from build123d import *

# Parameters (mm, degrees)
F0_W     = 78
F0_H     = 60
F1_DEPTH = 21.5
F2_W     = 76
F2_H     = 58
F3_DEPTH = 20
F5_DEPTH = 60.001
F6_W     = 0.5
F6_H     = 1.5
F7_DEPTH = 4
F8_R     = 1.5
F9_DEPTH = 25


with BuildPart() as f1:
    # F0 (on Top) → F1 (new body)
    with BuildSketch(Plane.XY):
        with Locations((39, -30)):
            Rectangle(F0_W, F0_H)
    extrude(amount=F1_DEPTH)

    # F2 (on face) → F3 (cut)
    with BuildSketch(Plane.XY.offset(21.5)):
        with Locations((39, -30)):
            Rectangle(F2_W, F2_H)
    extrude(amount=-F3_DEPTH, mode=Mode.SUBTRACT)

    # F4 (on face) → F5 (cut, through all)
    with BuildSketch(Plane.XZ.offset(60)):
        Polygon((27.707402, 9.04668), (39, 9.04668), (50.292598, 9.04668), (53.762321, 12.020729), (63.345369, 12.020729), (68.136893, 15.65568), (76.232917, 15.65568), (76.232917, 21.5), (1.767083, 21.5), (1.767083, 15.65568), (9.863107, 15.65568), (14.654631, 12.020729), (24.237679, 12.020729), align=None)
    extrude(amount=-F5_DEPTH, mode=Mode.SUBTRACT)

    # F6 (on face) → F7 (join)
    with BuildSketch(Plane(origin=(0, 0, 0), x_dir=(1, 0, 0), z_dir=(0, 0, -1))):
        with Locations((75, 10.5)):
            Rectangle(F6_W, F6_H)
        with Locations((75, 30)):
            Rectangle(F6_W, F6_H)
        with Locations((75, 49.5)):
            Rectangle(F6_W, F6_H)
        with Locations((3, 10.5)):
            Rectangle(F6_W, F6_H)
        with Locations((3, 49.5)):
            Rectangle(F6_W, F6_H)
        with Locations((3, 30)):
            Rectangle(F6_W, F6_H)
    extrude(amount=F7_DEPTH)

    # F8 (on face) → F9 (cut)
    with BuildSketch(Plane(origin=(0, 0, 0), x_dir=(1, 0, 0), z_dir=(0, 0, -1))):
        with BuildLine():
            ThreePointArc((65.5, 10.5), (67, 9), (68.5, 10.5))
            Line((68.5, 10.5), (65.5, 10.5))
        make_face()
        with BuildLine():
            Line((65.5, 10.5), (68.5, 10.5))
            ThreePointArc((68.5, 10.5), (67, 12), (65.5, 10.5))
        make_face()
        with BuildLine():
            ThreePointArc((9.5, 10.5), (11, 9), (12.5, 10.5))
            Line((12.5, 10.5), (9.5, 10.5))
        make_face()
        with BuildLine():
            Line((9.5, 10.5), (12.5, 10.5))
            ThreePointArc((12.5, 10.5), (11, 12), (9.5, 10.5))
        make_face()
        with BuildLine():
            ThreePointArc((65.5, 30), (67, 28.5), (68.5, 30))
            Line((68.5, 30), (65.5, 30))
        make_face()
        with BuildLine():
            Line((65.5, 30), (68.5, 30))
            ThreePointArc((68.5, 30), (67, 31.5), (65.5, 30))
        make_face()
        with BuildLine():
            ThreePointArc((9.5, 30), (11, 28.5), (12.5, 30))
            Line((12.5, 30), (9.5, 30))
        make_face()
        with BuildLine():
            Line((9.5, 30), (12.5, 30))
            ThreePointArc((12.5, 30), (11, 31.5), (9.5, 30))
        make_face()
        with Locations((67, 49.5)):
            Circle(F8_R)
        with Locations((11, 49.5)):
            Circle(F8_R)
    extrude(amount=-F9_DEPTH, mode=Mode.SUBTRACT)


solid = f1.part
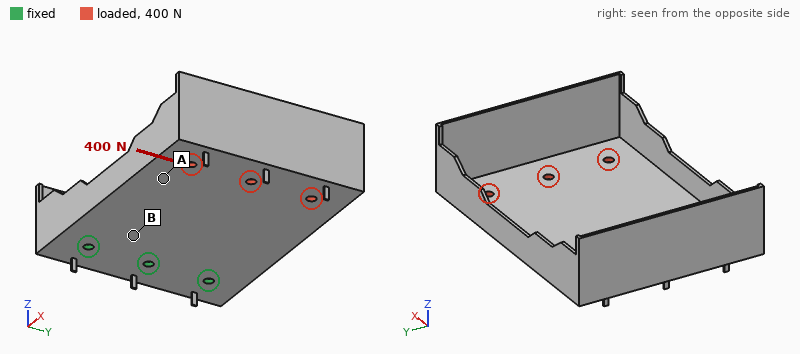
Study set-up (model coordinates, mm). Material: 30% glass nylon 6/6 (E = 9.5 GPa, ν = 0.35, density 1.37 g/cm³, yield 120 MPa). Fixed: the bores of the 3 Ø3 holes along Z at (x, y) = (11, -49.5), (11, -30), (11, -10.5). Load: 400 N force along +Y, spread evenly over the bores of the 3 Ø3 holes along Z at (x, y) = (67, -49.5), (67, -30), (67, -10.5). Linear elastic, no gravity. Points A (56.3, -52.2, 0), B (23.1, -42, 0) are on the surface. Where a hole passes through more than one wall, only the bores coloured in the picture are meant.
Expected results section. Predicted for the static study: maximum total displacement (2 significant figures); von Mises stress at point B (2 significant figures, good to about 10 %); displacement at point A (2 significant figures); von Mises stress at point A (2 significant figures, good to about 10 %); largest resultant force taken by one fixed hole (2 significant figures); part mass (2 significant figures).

0.40 mm
15 MPa
0.19 mm
5.7 MPa
570 N
15 g
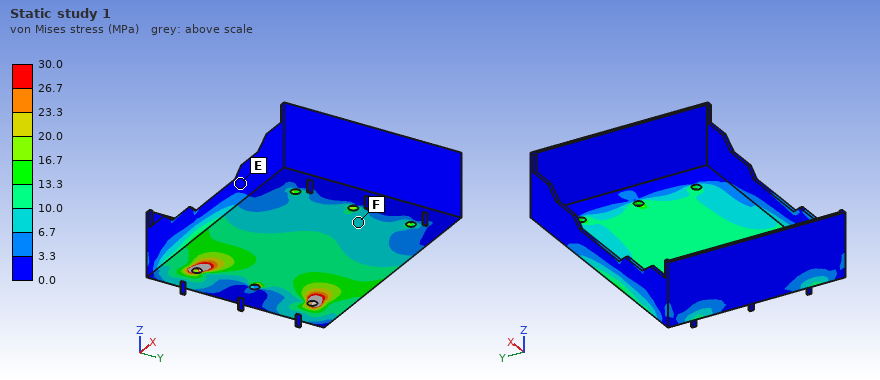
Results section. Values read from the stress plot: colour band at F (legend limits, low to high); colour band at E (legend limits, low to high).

6.7 to 10.0 MPa
0.0 to 3.3 MPa
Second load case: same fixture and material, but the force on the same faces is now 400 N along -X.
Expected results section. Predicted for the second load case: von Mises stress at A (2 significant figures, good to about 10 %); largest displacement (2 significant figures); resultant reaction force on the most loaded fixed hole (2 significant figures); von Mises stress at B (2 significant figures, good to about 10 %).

4.9 MPa
93 µm
140 N
4.6 MPa
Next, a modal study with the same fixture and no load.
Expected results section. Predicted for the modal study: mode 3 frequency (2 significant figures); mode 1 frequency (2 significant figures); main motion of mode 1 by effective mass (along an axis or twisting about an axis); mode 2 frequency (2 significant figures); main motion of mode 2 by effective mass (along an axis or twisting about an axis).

1100 Hz
200 Hz
along Z
310 Hz
twisting about X
